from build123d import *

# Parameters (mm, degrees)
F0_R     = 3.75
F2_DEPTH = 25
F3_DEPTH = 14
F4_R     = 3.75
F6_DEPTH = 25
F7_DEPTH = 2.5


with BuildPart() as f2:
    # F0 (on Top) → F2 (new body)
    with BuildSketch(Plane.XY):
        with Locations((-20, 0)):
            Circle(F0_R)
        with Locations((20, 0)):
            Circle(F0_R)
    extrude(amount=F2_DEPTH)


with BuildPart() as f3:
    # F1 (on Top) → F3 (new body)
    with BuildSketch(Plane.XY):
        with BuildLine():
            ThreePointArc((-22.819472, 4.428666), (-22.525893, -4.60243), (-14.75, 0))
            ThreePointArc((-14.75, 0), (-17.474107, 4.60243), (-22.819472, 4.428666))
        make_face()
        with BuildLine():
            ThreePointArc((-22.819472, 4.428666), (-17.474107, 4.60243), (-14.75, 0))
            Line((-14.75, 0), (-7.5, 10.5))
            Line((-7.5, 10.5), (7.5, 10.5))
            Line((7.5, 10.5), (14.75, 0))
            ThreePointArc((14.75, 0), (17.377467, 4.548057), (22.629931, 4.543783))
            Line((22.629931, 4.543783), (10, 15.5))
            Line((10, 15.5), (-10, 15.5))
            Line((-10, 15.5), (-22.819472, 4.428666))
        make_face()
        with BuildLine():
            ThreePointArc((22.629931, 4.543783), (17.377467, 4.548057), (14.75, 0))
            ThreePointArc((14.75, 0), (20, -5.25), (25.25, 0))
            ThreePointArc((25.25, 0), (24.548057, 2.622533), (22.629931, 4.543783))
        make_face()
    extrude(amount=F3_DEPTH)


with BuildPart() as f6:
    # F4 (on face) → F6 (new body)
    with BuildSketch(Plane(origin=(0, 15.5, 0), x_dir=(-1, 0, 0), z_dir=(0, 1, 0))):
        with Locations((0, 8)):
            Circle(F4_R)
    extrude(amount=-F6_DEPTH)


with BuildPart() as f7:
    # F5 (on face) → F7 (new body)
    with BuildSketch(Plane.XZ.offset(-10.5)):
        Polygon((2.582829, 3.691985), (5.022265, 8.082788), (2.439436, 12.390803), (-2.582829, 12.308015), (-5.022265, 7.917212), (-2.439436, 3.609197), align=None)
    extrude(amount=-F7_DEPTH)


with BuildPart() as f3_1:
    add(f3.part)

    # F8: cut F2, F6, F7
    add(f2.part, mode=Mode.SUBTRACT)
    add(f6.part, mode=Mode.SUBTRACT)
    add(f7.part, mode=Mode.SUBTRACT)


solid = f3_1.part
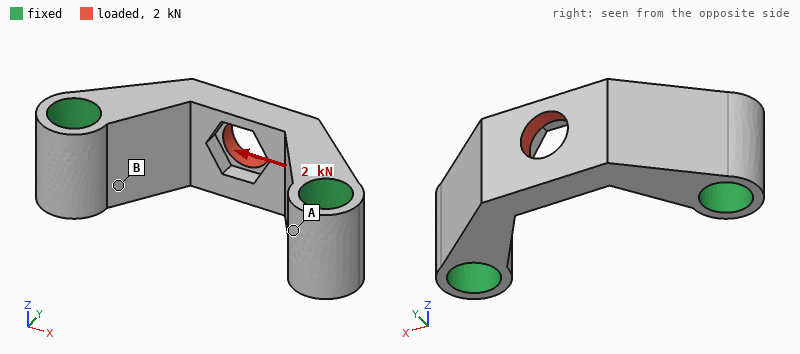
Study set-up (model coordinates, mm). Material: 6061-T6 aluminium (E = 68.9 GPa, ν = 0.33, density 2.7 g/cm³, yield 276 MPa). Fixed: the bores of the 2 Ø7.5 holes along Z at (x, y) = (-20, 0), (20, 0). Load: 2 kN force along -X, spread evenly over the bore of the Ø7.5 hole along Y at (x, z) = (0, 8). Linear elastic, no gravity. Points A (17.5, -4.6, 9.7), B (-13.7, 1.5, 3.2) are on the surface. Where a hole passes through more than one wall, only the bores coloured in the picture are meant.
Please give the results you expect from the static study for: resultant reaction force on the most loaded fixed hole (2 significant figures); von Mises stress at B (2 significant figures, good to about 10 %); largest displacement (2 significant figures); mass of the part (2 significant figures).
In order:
1.1 kN
16 MPa
13 µm
12 g
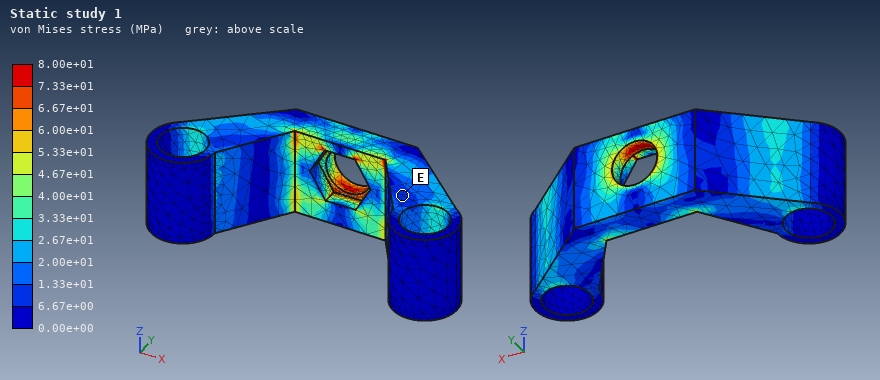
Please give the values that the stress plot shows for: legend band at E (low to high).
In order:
6.67e+00 to 1.33e+01 MPa
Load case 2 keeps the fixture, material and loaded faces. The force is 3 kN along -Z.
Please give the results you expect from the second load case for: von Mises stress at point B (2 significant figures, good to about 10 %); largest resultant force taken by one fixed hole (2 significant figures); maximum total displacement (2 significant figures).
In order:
31 MPa
1.5 kN
49 µm
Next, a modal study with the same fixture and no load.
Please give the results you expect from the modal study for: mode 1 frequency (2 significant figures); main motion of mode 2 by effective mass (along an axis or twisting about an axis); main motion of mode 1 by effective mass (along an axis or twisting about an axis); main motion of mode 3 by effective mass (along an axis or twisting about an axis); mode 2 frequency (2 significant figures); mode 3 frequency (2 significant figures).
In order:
27 kHz
along X
along Z
along Y
29 kHz
35 kHz
